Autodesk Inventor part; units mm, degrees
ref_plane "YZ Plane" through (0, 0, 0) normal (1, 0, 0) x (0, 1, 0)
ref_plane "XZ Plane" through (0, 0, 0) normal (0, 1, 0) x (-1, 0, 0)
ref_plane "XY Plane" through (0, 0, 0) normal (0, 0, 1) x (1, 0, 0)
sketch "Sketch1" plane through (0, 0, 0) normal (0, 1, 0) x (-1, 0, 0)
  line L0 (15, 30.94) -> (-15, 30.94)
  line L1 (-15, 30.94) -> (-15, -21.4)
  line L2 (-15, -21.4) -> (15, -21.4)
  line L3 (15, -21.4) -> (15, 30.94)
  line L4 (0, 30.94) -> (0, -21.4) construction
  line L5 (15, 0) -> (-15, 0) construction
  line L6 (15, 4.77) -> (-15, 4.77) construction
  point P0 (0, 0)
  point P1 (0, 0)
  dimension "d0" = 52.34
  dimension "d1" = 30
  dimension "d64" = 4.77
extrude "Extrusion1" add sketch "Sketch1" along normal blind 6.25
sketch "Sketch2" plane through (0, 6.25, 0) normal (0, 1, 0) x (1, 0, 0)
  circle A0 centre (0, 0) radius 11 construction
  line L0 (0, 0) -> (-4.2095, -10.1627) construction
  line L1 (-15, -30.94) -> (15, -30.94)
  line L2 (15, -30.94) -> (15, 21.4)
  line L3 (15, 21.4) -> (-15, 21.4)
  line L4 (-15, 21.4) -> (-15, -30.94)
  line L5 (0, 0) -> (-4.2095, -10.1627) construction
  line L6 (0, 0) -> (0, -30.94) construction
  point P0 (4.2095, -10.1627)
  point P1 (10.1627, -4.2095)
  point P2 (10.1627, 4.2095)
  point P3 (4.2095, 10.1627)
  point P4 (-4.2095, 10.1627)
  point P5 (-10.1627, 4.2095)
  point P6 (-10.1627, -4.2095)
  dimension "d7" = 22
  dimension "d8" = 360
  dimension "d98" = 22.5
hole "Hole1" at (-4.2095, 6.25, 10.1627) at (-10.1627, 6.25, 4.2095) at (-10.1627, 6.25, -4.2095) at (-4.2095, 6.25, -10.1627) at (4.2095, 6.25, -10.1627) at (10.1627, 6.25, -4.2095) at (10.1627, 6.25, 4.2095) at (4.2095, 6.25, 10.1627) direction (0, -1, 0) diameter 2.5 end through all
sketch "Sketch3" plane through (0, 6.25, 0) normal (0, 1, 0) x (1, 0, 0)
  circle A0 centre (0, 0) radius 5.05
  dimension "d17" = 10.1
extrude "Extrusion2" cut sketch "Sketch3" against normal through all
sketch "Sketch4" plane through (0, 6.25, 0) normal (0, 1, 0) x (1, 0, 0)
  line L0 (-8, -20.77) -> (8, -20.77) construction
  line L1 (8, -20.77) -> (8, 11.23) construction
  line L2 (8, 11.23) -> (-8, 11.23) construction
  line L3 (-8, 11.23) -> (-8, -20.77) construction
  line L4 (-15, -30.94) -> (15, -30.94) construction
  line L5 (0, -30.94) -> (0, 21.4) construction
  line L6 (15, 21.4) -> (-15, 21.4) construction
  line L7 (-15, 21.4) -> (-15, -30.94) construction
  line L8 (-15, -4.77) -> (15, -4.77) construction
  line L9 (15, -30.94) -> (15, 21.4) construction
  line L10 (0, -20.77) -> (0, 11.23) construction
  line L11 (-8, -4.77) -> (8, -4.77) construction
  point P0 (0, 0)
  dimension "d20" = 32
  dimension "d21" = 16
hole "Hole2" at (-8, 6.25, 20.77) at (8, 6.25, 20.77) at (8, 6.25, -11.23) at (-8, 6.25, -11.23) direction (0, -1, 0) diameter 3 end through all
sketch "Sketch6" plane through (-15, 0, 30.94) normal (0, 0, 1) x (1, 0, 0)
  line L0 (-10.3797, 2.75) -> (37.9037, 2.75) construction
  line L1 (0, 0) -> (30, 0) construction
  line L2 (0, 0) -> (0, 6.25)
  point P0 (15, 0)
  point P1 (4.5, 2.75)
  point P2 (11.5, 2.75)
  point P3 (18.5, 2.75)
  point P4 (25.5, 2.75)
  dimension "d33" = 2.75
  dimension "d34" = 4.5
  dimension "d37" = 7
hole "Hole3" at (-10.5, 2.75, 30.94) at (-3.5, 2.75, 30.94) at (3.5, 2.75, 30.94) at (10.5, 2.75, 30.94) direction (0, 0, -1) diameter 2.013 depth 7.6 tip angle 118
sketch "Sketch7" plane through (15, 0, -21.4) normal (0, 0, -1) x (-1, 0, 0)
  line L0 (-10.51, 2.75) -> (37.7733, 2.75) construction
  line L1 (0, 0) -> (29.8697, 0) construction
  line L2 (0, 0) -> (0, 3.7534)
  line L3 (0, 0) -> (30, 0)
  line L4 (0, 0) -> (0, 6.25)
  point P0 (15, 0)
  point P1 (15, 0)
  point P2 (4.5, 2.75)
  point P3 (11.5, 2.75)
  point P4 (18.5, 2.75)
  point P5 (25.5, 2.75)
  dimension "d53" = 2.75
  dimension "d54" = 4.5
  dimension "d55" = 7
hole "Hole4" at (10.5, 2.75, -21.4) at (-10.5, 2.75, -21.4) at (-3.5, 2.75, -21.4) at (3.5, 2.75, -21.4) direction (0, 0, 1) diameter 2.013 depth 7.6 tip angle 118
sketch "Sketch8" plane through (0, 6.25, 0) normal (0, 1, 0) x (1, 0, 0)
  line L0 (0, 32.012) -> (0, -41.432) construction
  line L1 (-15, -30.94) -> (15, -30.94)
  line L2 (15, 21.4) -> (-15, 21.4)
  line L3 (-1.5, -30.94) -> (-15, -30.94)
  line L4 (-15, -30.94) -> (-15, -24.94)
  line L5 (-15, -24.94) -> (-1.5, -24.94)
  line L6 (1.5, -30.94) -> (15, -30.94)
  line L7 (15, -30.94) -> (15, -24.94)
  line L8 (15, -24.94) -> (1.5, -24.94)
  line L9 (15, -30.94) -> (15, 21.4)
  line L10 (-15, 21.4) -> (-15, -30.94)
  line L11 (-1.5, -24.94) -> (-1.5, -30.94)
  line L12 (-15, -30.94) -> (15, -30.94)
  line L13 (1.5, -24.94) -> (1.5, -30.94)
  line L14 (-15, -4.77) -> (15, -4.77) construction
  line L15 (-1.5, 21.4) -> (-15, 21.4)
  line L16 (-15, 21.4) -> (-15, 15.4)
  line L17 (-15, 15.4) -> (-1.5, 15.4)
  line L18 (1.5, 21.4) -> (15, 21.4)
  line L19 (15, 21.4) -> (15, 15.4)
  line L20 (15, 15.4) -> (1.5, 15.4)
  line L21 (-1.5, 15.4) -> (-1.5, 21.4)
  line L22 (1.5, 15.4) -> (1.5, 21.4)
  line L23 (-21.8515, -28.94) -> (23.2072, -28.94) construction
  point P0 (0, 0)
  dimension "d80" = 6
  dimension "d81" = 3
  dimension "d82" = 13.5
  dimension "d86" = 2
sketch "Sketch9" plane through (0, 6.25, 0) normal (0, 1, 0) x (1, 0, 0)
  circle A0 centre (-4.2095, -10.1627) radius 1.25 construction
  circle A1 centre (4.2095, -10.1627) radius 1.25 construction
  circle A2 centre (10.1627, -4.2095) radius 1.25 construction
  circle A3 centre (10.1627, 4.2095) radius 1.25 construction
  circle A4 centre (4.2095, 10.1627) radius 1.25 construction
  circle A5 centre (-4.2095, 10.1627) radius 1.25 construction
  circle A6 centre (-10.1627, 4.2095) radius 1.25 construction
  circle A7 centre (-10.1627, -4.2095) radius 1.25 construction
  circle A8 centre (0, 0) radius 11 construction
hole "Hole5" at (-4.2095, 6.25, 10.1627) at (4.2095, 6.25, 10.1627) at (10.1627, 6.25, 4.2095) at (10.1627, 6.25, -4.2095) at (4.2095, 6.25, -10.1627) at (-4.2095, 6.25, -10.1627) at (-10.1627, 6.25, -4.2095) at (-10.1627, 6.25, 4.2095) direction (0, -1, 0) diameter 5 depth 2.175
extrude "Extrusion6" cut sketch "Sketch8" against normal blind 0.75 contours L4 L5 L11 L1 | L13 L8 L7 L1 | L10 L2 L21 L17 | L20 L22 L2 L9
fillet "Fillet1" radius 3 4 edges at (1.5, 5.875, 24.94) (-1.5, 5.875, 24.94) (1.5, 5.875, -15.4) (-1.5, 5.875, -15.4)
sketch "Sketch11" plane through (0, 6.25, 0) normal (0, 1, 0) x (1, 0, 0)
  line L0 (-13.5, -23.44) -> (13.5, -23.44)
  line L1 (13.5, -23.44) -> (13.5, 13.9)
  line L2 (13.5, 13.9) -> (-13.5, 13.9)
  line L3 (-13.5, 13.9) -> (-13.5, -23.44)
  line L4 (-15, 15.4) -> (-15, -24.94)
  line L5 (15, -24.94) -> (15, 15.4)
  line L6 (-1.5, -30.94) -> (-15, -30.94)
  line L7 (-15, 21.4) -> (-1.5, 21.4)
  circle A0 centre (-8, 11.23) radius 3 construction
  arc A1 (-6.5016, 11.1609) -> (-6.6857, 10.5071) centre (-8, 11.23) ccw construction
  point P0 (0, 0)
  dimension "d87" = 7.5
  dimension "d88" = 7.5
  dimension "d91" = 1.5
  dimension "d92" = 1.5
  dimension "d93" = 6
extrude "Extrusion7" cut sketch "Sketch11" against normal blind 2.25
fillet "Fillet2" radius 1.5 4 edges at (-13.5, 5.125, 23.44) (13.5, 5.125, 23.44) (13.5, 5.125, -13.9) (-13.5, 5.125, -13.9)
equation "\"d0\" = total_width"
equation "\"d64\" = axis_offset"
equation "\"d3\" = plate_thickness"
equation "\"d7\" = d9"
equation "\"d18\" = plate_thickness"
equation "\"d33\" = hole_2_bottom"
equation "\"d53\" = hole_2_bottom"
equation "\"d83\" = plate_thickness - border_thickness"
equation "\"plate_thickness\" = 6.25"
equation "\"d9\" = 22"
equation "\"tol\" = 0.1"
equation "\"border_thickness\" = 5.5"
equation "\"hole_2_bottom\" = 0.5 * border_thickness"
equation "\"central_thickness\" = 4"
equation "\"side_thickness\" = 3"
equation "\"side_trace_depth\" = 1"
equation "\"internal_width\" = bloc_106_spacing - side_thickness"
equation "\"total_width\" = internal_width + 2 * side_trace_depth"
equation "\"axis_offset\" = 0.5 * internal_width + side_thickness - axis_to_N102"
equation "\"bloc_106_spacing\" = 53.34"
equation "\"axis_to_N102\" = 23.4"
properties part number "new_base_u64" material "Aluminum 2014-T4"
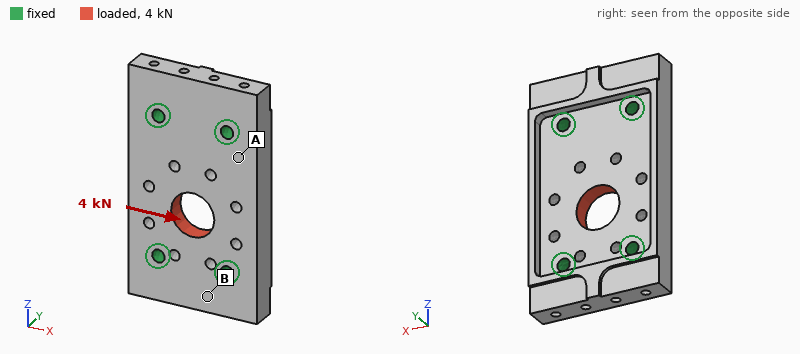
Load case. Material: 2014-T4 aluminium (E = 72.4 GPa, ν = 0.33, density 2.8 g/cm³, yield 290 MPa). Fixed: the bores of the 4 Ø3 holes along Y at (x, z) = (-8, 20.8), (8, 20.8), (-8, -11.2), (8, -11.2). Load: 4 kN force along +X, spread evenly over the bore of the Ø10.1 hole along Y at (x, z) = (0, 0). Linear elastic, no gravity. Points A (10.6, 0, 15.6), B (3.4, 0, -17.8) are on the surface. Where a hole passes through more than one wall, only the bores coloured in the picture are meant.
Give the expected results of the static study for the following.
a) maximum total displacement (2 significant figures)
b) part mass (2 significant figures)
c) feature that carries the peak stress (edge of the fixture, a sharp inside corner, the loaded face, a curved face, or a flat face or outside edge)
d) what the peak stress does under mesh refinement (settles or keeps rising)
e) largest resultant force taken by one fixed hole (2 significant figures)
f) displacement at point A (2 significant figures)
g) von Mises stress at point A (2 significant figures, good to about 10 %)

14 µm
18 g
edge of the fixture
keeps rising
1.3 kN
4.1 µm
17 MPa
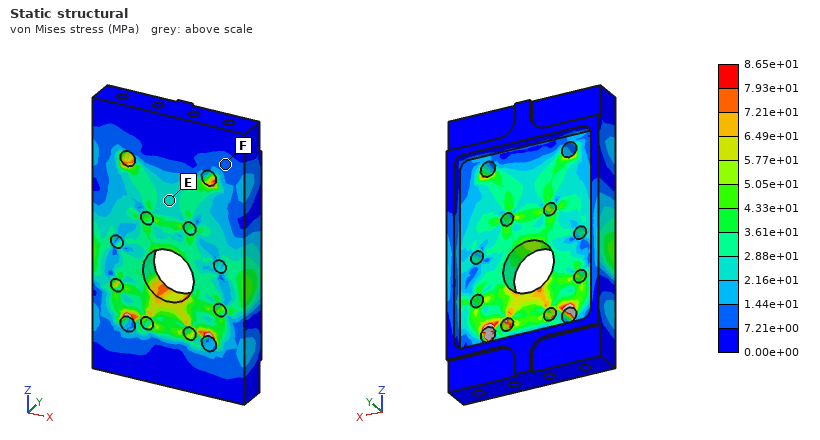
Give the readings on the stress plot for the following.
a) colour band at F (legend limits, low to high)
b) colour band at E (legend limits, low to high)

7.21e+00 to 1.44e+01 MPa
2.16e+01 to 2.88e+01 MPa
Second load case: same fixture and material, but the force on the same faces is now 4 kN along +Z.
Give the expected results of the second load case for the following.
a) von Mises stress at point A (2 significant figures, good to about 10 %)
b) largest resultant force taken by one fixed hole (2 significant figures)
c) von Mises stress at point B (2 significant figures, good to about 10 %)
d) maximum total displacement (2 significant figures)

13 MPa
1.2 kN
13 MPa
6.2 µm
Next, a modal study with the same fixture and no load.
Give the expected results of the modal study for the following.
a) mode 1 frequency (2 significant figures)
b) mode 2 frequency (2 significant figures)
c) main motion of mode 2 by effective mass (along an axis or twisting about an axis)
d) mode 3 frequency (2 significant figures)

18 kHz
21 kHz
twisting about Z
24 kHz
